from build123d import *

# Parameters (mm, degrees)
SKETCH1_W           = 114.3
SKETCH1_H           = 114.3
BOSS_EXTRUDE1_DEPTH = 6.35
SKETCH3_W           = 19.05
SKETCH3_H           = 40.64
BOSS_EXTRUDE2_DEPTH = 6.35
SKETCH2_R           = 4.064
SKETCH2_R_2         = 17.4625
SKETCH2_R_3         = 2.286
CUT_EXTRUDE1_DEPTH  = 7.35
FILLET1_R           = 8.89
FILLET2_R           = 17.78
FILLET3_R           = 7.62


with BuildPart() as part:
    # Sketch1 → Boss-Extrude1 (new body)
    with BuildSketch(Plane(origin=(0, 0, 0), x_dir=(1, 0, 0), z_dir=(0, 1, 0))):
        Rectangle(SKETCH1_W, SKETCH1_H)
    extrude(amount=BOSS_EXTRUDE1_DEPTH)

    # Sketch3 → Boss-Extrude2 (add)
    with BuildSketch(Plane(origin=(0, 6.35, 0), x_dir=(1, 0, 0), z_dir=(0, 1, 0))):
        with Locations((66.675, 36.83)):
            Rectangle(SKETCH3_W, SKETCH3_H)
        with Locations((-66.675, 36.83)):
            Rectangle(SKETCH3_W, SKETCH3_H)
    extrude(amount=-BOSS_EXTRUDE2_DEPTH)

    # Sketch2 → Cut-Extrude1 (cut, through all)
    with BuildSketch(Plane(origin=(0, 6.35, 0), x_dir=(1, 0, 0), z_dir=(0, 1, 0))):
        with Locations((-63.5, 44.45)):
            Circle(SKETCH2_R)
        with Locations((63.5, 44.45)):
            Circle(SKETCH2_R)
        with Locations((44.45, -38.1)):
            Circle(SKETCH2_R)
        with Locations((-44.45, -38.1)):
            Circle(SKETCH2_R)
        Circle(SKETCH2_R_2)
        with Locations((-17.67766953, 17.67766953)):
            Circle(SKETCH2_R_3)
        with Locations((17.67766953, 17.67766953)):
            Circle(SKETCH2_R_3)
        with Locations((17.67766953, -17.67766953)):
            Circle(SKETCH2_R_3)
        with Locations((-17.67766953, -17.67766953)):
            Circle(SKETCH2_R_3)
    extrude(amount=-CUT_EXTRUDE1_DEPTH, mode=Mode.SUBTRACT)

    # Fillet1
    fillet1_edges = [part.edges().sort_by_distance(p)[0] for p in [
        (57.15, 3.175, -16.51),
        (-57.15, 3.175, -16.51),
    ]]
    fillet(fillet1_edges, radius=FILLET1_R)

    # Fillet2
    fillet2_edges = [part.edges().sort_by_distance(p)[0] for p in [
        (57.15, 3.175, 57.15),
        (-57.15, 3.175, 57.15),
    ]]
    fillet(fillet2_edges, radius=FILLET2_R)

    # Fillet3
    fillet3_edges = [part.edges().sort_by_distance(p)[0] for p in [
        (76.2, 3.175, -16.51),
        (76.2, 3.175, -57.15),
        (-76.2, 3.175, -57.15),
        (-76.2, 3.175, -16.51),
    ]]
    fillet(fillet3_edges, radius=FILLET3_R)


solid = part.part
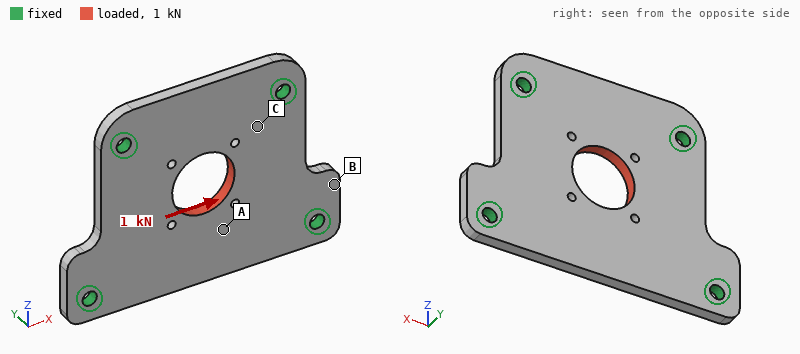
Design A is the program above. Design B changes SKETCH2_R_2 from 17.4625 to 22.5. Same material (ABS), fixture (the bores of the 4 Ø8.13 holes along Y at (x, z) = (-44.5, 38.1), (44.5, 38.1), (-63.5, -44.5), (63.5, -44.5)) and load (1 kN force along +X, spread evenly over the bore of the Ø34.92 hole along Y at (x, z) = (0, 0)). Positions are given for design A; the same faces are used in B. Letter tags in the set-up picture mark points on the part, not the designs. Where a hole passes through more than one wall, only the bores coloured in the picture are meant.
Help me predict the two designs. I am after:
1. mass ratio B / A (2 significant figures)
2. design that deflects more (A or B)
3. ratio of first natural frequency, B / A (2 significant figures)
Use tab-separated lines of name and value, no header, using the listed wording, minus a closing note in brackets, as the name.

mass ratio B / A	0.95
design that deflects more	B
ratio of first natural frequency, B / A	1.0
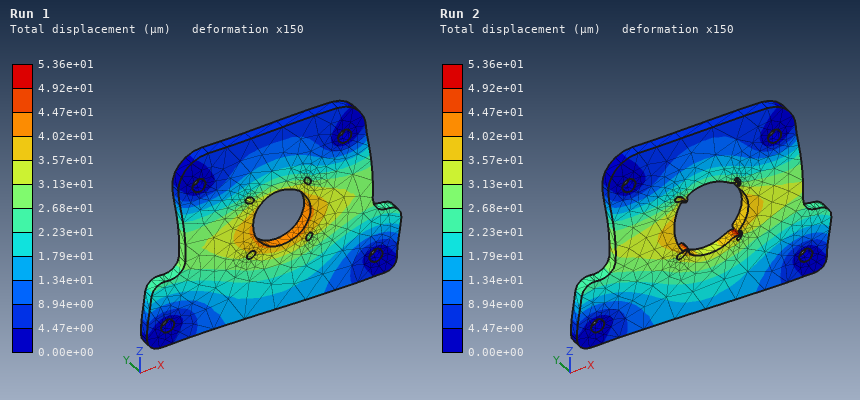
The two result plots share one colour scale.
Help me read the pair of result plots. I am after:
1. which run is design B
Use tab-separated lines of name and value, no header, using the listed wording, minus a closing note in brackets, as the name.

which run is design B	Run 2
